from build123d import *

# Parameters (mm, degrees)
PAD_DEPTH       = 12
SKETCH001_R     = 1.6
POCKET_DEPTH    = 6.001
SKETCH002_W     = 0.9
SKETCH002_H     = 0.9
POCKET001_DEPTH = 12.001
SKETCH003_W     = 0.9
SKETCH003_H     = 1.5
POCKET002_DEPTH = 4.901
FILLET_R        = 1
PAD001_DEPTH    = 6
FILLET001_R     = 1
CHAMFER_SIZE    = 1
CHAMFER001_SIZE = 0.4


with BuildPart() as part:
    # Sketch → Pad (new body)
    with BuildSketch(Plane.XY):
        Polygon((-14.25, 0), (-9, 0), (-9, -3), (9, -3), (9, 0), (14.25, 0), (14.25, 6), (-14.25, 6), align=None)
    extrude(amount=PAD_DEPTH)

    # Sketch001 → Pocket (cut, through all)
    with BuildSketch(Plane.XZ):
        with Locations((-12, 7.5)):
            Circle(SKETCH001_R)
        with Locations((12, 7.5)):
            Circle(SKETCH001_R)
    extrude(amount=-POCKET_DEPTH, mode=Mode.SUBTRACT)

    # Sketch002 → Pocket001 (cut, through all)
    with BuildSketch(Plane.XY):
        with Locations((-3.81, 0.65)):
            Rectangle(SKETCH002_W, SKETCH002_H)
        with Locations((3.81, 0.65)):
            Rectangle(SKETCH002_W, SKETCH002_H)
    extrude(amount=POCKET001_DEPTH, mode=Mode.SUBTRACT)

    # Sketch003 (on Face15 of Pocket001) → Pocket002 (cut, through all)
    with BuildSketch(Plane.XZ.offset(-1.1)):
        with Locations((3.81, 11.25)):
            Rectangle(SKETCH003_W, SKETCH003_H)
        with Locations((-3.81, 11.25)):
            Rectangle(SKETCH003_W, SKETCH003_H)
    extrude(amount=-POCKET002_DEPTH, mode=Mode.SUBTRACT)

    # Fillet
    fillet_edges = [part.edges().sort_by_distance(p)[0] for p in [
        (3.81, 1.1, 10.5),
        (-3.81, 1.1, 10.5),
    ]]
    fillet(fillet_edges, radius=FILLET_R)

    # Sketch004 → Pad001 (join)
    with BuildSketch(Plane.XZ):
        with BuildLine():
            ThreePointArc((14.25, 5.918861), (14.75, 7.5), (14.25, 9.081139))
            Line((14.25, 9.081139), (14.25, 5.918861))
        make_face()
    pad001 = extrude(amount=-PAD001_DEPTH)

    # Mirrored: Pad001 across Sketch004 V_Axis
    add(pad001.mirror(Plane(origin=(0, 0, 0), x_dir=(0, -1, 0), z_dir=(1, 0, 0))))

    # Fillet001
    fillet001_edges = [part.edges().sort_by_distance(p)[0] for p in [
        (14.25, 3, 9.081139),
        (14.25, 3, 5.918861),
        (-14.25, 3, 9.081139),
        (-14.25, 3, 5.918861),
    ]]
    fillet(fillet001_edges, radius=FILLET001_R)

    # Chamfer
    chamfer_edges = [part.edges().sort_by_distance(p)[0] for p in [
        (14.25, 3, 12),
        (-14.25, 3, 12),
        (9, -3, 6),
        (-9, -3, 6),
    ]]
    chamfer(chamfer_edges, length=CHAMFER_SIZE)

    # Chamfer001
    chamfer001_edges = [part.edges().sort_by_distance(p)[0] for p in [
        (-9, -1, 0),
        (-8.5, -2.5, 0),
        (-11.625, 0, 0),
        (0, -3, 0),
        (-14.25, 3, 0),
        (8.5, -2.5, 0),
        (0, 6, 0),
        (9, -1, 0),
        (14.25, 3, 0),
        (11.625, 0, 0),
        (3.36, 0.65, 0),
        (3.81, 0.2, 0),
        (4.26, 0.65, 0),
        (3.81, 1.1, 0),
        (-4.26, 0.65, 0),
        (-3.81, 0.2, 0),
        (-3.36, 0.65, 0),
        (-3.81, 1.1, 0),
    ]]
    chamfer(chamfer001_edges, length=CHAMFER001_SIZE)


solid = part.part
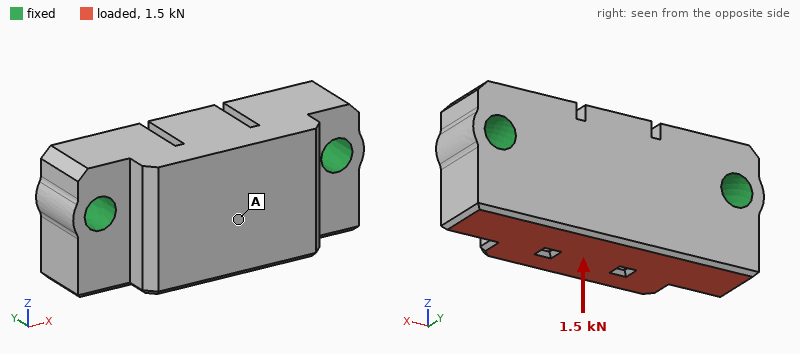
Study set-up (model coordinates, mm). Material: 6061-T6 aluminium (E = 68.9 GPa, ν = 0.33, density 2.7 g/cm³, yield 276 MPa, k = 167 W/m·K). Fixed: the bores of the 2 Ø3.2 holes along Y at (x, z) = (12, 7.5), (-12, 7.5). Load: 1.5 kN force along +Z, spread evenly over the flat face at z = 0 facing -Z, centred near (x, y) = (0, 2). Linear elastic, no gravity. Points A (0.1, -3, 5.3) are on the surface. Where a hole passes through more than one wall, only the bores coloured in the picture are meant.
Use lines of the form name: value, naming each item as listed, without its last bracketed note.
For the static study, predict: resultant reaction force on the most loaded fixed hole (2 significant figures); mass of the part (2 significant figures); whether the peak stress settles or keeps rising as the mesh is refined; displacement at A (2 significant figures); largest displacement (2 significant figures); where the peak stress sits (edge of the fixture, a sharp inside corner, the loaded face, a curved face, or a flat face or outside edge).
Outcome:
resultant reaction force on the most loaded fixed hole: 790 N
mass of the part: 6.9 g
whether the peak stress settles or keeps rising as the mesh is refined: keeps rising
displacement at A: 5.4 µm
largest displacement: 5.9 µm
where the peak stress sits: edge of the fixture
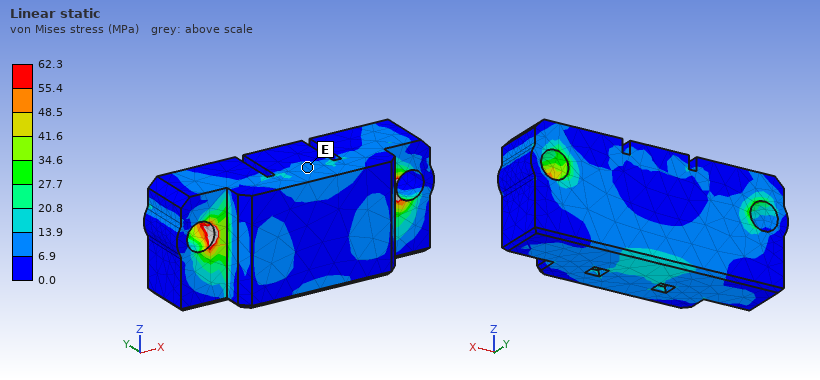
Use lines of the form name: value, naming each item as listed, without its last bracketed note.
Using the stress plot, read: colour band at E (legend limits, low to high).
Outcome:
colour band at E: 6.9 to 13.9 MPa
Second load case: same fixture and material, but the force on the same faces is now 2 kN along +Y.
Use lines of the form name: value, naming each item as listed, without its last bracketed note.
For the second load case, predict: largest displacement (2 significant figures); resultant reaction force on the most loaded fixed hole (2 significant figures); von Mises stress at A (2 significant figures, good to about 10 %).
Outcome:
largest displacement: 27 µm
resultant reaction force on the most loaded fixed hole: 1.0 kN
von Mises stress at A: 28 MPa
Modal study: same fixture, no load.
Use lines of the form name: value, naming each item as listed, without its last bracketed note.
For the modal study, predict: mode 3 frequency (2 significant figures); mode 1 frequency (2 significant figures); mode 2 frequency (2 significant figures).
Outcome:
mode 3 frequency: 47 kHz
mode 1 frequency: 32 kHz
mode 2 frequency: 40 kHz
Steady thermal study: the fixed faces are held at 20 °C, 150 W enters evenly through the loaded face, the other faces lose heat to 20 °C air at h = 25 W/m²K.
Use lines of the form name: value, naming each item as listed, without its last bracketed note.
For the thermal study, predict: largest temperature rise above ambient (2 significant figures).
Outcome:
largest temperature rise above ambient: 57 K
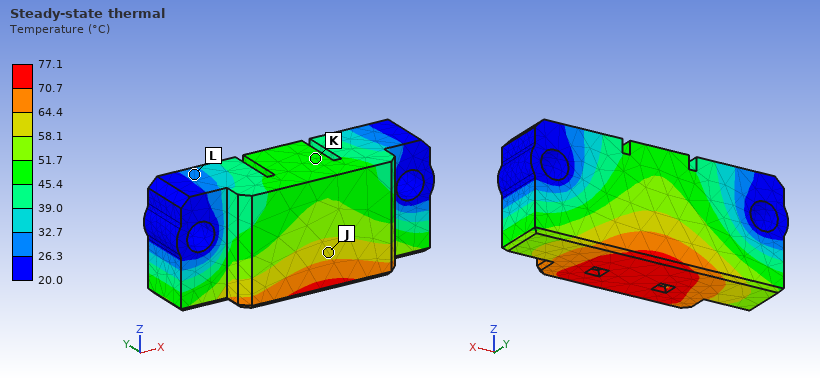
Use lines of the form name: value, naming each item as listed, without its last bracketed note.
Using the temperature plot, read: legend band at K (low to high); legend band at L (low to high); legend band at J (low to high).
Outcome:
legend band at K: 45.4 to 51.7 °C
legend band at L: 26.3 to 32.7 °C
legend band at J: 58.1 to 64.4 °C
